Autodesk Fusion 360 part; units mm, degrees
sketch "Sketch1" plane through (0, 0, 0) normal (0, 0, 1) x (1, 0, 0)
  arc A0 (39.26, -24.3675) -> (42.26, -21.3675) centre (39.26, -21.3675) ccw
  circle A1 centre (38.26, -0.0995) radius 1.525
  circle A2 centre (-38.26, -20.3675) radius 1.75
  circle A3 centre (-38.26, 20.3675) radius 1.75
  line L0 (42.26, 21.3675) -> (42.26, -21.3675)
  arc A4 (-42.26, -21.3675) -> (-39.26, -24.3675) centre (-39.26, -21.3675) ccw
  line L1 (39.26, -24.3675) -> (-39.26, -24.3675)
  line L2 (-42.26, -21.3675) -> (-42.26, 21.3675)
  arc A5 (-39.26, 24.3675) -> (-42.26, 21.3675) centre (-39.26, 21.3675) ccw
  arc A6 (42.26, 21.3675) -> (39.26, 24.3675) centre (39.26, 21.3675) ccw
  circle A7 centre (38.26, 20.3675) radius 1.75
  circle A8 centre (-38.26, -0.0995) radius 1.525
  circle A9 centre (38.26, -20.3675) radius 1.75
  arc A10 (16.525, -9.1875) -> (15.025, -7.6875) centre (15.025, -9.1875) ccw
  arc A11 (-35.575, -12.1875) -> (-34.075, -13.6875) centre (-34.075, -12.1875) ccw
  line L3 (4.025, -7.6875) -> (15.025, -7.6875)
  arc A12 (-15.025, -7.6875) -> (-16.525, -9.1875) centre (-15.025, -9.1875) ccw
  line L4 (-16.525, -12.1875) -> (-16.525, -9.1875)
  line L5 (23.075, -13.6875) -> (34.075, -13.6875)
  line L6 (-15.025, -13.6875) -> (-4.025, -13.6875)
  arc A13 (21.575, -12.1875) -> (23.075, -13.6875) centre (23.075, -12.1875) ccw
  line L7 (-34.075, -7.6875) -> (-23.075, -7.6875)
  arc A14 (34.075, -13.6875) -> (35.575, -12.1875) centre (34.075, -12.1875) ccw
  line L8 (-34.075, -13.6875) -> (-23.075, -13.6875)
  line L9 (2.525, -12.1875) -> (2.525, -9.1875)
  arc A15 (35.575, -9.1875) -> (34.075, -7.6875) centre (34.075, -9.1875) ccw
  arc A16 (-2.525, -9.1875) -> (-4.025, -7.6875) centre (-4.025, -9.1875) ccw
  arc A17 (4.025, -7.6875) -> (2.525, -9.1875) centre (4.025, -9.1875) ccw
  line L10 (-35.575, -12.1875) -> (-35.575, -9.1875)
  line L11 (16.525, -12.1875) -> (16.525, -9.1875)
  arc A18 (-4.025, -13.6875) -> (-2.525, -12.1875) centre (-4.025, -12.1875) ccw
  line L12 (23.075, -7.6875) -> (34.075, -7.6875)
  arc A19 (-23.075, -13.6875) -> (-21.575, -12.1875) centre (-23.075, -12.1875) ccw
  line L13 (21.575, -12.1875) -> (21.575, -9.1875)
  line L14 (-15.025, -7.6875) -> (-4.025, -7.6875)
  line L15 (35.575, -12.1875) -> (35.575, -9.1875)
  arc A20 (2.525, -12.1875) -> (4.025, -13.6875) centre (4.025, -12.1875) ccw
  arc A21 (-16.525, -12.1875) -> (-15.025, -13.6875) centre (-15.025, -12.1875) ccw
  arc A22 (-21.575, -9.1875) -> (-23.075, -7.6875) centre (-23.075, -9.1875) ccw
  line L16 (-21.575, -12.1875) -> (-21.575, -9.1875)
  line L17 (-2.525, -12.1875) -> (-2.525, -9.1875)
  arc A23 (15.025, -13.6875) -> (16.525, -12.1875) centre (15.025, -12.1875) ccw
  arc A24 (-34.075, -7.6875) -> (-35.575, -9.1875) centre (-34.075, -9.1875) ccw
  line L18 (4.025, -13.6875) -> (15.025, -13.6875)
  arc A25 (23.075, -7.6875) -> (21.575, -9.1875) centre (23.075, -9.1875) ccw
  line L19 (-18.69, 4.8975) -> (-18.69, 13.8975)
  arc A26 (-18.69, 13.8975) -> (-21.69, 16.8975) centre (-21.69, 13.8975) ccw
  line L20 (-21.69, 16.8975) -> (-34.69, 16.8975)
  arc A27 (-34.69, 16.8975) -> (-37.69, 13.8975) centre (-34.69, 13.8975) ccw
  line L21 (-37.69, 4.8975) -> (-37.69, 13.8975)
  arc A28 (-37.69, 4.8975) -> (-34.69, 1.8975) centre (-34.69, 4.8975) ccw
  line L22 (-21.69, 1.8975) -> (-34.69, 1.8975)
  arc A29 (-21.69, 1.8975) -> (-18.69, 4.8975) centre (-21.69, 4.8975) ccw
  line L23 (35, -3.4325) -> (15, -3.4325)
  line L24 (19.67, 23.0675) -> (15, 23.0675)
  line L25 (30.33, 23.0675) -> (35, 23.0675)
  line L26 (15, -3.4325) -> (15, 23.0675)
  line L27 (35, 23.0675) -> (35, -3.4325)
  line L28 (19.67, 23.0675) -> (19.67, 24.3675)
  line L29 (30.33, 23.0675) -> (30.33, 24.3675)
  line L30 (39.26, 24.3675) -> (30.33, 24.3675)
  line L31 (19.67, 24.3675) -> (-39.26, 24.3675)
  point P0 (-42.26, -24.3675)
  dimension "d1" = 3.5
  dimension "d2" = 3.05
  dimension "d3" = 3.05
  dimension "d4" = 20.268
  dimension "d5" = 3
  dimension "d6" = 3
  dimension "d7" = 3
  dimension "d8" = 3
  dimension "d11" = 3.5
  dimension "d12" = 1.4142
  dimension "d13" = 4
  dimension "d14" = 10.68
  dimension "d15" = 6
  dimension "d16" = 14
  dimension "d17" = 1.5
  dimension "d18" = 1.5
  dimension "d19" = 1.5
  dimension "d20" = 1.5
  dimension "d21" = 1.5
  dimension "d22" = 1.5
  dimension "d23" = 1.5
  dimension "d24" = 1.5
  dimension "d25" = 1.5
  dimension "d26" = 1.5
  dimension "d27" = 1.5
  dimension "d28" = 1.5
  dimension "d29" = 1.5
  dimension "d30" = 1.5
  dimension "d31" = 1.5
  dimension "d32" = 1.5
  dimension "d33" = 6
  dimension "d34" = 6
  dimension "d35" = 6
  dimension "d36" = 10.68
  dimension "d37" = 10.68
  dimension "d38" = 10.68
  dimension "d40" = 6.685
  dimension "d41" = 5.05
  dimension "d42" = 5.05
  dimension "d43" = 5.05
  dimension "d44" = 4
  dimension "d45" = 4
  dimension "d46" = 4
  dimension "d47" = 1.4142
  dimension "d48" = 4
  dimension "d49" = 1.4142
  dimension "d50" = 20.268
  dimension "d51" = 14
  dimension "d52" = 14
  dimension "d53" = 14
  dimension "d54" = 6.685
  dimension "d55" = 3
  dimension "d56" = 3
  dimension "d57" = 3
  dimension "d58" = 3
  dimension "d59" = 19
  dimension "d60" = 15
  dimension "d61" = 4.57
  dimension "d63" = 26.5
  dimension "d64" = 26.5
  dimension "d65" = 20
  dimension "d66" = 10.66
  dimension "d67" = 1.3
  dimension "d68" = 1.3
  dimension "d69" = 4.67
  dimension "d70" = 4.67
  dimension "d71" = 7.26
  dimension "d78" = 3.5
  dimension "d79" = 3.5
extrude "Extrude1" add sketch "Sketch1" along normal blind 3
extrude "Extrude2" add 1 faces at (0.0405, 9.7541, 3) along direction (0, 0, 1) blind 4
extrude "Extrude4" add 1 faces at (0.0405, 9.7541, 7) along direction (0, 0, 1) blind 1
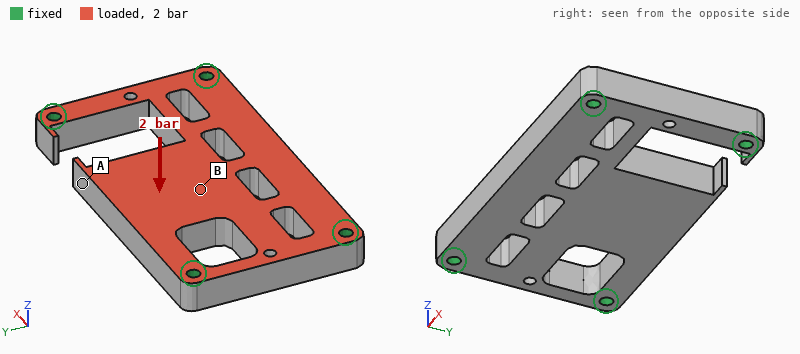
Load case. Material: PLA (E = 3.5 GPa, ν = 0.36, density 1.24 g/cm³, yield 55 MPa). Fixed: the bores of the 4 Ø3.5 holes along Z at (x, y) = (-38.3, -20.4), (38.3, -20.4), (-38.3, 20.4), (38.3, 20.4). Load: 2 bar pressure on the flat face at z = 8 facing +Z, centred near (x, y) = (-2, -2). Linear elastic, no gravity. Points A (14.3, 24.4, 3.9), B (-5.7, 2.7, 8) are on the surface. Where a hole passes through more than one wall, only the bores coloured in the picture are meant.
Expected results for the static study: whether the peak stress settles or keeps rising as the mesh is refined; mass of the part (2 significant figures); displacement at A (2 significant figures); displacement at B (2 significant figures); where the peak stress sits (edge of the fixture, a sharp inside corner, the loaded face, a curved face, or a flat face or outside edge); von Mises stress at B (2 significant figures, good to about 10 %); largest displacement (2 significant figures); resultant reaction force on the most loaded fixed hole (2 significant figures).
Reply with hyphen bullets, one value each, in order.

- keeps rising
- 29 g
- 0.70 mm
- 0.34 mm
- edge of the fixture
- 5.7 MPa
- 0.76 mm
- 200 N
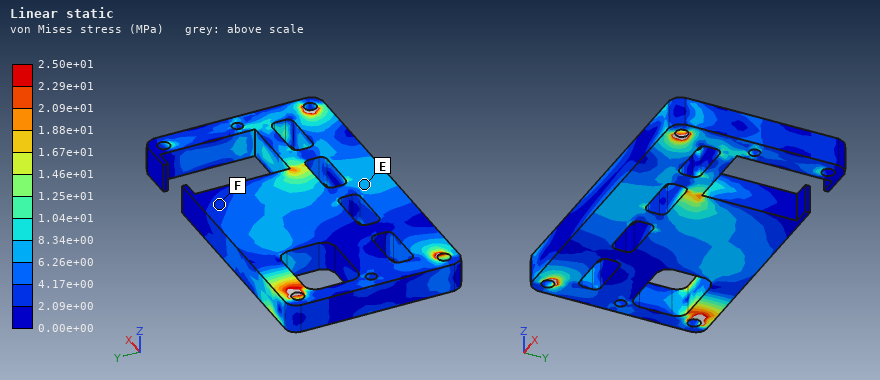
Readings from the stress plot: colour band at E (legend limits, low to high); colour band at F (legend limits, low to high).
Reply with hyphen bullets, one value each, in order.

- 6.26e+00 to 8.34e+00 MPa
- 2.09e+00 to 4.17e+00 MPa
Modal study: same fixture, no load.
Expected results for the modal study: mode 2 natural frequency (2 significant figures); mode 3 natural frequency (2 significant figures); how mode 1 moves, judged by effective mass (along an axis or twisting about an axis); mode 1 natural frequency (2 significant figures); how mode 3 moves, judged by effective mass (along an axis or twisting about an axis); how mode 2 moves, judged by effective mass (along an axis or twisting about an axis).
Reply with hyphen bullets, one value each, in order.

- 2200 Hz
- 2600 Hz
- along Z
- 1200 Hz
- along Y
- along Z
